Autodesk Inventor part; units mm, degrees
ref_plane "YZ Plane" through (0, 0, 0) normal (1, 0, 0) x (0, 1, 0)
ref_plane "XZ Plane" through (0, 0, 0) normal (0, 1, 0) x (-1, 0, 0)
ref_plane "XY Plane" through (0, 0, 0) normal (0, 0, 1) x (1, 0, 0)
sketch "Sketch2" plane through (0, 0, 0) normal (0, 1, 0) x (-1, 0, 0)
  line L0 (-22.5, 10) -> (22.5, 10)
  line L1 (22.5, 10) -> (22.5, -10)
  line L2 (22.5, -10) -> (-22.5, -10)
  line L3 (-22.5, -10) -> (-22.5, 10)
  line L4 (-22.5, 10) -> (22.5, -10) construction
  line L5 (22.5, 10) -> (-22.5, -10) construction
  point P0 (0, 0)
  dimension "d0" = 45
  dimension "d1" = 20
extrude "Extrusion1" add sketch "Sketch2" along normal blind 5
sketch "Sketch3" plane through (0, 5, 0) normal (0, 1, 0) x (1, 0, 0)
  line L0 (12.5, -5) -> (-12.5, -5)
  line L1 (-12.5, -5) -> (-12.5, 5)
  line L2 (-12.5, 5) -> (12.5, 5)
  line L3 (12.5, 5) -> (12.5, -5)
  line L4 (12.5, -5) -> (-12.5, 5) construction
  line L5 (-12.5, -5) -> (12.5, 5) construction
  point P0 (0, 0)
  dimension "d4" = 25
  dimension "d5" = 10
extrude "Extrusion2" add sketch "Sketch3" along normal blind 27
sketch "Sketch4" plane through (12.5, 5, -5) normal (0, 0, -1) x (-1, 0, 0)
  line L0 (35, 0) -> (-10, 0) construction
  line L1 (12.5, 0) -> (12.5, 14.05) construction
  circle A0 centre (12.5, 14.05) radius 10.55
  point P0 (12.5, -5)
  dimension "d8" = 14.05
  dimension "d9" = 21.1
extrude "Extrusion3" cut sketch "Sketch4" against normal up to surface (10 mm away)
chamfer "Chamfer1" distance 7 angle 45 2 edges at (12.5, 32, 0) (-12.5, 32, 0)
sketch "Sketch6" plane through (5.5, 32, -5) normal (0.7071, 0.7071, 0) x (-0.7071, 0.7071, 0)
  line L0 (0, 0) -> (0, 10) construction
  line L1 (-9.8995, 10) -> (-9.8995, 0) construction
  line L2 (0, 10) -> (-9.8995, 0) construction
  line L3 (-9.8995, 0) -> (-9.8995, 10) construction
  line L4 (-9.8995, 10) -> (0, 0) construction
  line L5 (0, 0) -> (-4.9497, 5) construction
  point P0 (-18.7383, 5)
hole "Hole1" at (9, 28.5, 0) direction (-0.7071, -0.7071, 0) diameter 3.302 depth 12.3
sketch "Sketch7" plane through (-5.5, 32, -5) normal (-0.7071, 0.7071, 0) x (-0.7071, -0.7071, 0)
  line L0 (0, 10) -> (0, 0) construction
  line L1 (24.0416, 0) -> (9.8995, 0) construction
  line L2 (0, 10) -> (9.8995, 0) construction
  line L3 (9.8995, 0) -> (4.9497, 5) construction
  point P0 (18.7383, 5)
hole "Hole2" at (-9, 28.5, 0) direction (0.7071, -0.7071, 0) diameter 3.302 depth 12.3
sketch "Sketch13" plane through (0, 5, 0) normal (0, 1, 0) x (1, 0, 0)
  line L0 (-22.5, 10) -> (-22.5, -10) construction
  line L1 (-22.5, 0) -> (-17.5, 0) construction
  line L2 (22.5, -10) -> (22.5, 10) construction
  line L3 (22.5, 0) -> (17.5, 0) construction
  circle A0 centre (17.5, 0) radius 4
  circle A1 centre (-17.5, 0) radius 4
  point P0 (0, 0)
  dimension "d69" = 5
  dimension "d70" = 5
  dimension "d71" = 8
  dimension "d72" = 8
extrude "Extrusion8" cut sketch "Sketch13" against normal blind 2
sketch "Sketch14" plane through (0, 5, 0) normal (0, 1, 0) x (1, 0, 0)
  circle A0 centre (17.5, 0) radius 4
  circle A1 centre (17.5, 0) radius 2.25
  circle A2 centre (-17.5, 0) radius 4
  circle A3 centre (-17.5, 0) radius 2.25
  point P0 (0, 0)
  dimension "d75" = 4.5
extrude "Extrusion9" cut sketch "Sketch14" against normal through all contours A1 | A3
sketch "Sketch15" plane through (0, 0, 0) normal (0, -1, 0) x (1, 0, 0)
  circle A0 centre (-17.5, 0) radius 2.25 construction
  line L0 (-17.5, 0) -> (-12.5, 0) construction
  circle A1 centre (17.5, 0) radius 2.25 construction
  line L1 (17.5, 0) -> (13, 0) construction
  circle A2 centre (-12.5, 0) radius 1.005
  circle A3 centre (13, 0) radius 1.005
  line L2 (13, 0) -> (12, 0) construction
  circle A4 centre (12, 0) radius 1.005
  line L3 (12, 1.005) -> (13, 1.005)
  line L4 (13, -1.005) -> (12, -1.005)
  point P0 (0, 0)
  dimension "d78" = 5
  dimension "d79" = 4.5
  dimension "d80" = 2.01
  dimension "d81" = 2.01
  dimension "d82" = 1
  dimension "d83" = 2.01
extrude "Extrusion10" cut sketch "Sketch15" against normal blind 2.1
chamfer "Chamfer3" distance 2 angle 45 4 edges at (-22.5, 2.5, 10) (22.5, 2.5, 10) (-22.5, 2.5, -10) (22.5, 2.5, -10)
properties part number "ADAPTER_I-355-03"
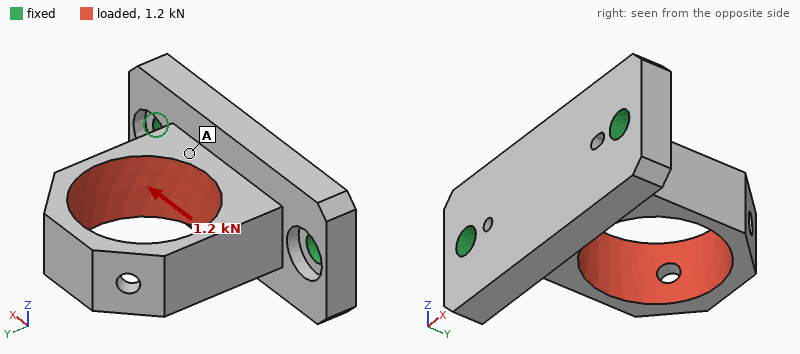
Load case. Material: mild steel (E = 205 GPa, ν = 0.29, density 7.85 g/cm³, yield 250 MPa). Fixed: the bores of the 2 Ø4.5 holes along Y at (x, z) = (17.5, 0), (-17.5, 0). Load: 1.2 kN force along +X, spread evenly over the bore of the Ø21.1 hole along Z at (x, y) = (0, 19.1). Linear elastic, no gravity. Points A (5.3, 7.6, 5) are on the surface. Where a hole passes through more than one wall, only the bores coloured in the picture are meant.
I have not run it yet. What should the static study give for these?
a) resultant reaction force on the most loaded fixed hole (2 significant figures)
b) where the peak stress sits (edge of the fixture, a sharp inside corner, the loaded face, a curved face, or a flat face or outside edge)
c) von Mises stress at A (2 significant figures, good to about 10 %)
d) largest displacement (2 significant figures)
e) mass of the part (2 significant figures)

900 N
the loaded face
27 MPa
47 µm
54 g
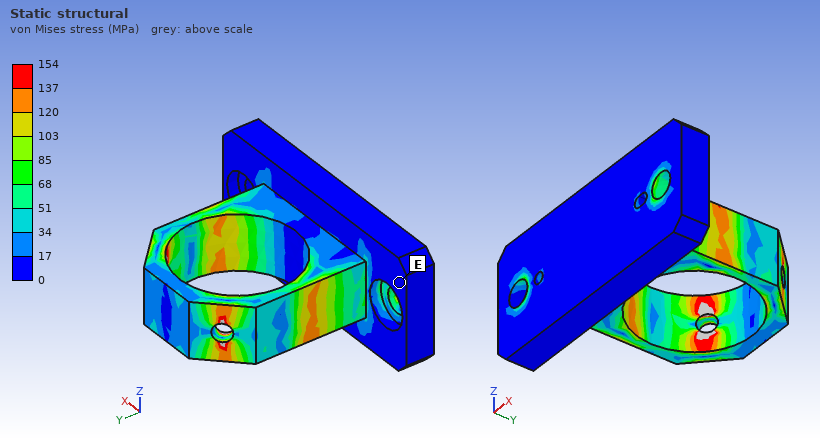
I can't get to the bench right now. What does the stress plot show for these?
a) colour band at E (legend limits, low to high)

0 to 17 MPa
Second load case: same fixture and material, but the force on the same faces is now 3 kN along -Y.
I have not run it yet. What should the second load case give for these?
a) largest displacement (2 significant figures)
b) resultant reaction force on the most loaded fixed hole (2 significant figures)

20 µm
1.7 kN
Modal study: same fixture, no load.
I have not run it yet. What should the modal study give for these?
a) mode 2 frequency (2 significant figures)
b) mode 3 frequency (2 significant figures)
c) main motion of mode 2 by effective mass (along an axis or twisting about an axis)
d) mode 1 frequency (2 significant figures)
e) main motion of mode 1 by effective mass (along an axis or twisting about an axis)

7000 Hz
15 kHz
along X
5000 Hz
along Z
